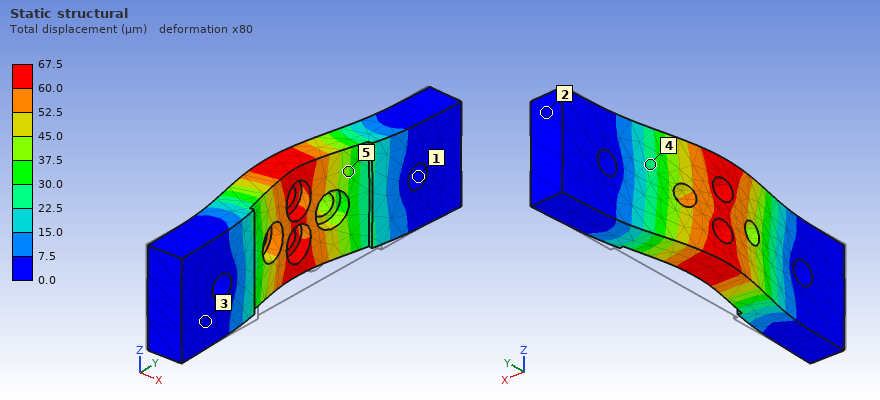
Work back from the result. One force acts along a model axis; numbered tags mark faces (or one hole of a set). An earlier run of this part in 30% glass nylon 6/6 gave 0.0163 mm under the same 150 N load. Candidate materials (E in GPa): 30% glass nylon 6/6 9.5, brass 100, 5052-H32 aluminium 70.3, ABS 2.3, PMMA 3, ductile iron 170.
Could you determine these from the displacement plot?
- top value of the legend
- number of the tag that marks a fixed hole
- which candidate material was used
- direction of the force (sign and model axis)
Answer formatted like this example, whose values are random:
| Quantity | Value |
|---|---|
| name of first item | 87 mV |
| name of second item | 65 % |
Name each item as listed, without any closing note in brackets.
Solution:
| Quantity | Value |
|---|---|
| top value of the legend | 67.5 µm |
| number of the tag that marks a fixed hole | 1 |
| which candidate material was used | ABS |
| direction of the force | -X |
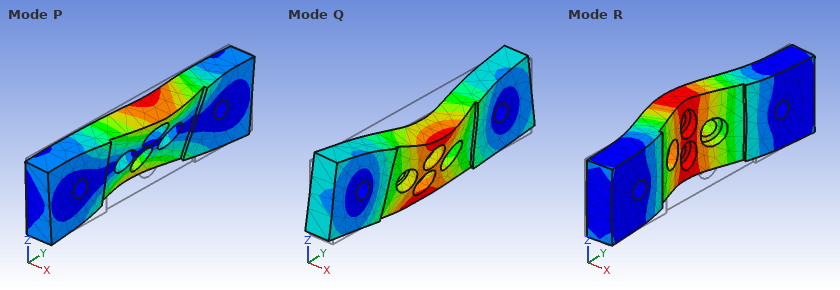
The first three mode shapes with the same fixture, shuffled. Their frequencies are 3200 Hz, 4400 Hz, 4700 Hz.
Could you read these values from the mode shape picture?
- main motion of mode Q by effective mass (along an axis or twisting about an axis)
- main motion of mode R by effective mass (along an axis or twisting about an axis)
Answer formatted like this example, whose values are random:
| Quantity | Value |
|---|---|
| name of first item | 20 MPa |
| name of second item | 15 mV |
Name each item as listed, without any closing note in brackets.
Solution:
| Quantity | Value |
|---|---|
| main motion of mode Q by effective mass | along Z |
| main motion of mode R by effective mass | along X |
